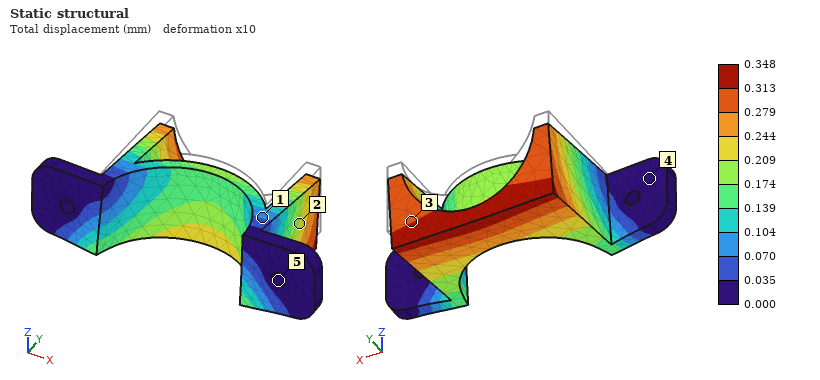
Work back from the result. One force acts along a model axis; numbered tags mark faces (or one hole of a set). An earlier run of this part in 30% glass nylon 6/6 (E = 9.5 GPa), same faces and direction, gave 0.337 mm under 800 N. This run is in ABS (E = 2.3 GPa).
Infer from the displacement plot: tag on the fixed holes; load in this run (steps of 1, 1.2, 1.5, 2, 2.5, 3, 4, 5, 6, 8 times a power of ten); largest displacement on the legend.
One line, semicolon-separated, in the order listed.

5; 200 N; 0.348 mm
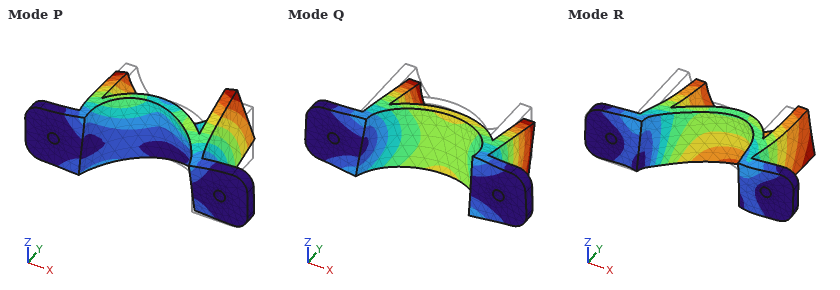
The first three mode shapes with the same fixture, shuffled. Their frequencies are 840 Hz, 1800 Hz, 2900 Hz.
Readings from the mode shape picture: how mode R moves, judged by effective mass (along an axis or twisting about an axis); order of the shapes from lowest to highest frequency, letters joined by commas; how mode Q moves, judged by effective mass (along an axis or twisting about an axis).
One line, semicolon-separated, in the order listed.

along X; Q, P, R; along Z
